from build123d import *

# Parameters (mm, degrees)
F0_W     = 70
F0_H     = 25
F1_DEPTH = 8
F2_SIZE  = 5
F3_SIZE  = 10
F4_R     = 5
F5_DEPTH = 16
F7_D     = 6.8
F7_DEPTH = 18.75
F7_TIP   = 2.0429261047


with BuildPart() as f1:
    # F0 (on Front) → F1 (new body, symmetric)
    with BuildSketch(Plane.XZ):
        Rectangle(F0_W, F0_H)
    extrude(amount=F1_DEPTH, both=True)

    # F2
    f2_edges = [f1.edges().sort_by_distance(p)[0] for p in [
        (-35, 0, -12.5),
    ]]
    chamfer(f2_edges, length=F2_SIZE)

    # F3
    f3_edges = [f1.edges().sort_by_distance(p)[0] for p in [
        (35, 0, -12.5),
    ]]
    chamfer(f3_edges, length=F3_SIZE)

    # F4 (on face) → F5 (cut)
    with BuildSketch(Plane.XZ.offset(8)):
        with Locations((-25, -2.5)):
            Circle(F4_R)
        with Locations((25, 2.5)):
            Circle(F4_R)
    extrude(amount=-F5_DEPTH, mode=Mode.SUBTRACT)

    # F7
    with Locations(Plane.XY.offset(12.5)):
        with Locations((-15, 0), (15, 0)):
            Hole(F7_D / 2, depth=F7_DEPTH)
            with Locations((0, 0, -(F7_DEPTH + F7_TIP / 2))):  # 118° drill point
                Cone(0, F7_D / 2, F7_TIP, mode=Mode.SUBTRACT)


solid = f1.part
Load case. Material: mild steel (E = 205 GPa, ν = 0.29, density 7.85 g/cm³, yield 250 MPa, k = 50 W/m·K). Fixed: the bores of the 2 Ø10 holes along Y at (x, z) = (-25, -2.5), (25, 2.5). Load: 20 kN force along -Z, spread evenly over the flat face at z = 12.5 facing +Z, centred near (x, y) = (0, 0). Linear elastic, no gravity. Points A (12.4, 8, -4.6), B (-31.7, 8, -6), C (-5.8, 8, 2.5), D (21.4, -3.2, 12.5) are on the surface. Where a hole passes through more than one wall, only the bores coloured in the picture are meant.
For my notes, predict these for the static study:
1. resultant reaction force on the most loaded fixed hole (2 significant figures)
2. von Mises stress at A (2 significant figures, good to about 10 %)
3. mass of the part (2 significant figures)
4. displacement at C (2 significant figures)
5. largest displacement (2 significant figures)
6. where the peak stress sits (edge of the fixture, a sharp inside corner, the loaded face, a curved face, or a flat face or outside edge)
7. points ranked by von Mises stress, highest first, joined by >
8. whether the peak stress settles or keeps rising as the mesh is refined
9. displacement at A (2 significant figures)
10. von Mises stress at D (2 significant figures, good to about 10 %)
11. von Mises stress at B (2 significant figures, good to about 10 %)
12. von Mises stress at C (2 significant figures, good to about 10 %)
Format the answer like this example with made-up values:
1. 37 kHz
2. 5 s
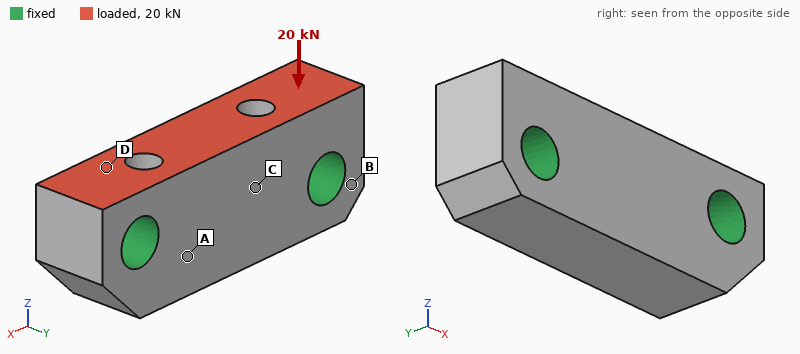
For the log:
1. 10 kN
2. 26 MPa
3. 180 g
4. 4.5 µm
5. 5.4 µm
6. edge of the fixture
7. D > A > C > B
8. keeps rising
9. 3.0 µm
10. 38 MPa
11. 6.5 MPa
12. 17 MPa
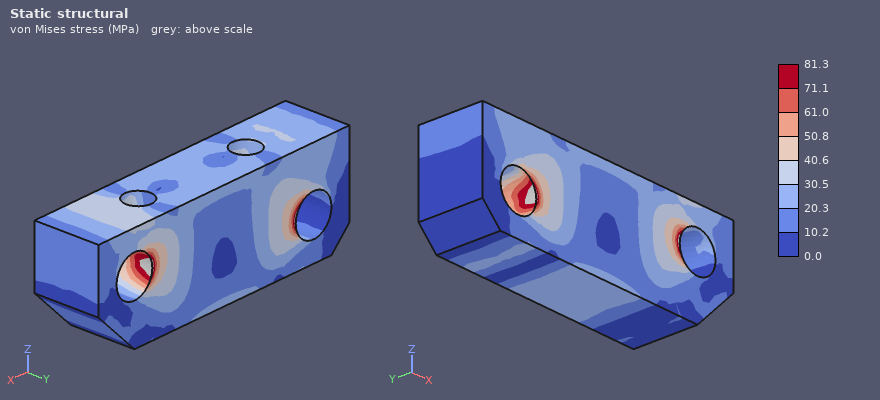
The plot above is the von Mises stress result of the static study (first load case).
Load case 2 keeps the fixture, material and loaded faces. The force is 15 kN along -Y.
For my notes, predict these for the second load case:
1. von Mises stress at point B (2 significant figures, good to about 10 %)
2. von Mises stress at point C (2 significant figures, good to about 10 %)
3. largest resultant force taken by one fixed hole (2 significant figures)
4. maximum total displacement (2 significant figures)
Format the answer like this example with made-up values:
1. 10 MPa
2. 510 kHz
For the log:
1. 14 MPa
2. 36 MPa
3. 7.6 kN
4. 16 µm
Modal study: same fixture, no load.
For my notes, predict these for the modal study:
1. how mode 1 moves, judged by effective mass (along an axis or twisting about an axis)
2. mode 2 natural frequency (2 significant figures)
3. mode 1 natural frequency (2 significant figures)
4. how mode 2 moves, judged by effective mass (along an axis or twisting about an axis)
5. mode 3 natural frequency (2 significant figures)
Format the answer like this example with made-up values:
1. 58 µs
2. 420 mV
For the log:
1. along Y
2. 24 kHz
3. 20 kHz
4. along Z
5. 27 kHz
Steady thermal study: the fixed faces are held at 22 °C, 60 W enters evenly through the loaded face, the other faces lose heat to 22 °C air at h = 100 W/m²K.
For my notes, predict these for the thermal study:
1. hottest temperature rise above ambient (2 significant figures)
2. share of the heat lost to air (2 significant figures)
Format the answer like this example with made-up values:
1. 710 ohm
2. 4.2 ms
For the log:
1. 23 K
2. 6.7 %
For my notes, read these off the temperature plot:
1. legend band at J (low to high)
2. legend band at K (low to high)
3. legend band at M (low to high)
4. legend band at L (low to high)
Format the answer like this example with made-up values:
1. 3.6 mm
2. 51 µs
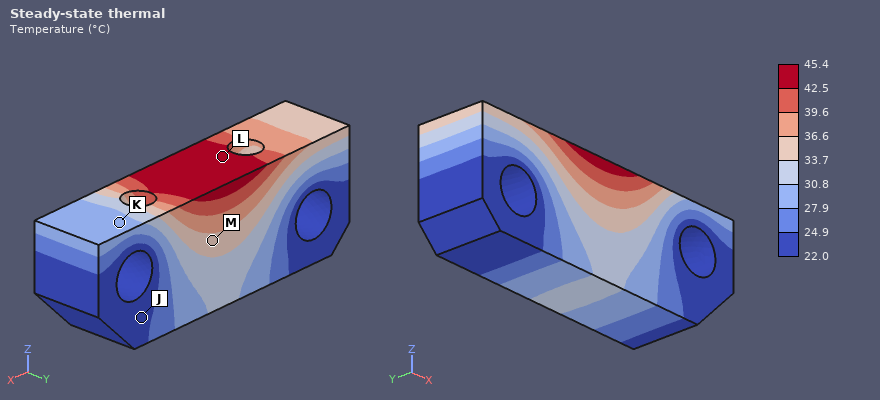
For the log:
1. 22.0 to 24.9 °C
2. 27.9 to 30.8 °C
3. 33.7 to 36.6 °C
4. 42.5 to 45.4 °C
